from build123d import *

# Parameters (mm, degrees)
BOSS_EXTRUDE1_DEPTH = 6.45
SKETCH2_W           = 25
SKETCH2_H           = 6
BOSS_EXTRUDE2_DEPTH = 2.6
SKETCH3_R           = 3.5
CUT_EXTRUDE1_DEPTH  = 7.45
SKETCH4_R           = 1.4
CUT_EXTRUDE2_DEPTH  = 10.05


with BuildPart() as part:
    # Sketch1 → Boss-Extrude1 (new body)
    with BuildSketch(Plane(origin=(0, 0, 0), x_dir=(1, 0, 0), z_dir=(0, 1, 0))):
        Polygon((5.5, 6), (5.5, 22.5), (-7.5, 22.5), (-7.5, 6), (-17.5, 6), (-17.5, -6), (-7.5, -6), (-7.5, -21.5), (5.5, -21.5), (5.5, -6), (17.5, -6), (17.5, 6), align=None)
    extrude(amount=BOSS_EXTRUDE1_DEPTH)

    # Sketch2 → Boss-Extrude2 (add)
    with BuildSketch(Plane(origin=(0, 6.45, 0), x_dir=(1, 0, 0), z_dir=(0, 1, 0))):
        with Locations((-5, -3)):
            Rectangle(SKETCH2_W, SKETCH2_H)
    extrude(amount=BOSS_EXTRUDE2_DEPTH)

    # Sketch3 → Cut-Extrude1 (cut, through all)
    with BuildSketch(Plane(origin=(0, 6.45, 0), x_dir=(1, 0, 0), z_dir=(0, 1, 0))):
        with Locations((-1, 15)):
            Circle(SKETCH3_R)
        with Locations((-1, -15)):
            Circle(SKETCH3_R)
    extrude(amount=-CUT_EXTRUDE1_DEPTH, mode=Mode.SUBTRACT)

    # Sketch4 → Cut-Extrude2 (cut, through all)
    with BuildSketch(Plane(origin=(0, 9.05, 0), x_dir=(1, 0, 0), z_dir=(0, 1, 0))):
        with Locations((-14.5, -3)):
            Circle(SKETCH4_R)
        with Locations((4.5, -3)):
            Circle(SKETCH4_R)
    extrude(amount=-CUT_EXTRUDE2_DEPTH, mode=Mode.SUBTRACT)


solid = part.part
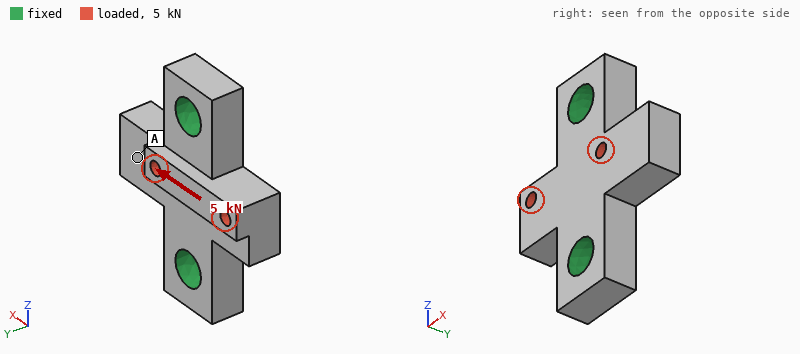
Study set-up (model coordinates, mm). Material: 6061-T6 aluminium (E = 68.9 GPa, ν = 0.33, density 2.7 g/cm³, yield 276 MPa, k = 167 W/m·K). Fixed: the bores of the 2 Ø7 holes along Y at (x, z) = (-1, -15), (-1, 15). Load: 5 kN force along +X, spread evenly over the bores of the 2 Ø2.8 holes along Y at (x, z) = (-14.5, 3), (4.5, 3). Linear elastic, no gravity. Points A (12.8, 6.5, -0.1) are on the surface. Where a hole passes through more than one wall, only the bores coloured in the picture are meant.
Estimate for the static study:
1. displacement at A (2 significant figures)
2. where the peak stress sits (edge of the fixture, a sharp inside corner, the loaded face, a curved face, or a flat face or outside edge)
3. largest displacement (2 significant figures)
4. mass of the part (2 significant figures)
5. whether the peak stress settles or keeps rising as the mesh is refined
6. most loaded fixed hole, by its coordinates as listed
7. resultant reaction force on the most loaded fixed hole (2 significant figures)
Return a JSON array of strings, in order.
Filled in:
["25 µm", "edge of the fixture", "41 µm", "14 g", "keeps rising", "(-1, 15)", "3.2 kN"]
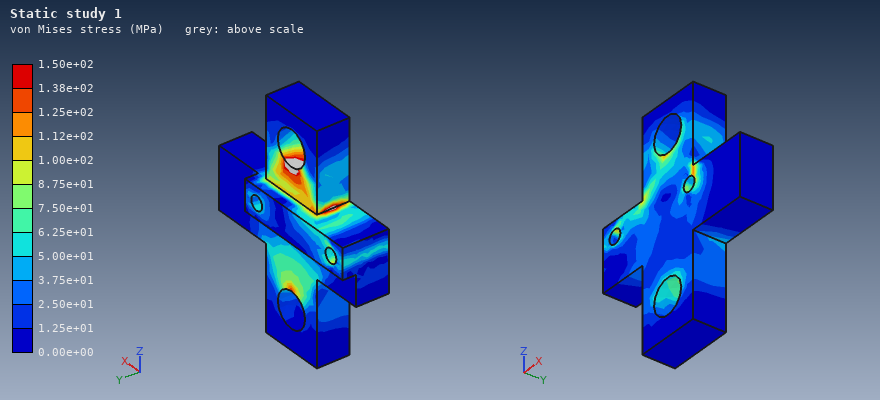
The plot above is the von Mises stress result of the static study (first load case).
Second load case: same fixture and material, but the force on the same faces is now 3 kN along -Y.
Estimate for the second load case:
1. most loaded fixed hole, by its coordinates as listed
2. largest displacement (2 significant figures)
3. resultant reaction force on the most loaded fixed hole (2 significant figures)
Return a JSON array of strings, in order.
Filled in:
["(-1, 15)", "96 µm", "2.0 kN"]
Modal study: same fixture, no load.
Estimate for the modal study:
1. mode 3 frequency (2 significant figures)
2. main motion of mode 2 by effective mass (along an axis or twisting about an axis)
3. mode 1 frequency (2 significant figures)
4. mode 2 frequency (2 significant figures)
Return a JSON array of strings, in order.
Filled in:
["29 kHz", "along Y", "12 kHz", "18 kHz"]
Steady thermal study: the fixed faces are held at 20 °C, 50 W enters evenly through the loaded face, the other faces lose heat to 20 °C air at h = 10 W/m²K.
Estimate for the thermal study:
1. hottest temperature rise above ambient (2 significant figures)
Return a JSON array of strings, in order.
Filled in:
["36 K"]
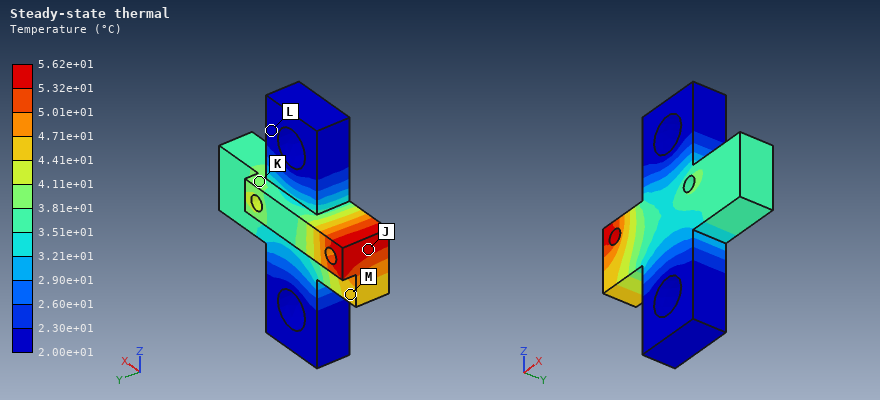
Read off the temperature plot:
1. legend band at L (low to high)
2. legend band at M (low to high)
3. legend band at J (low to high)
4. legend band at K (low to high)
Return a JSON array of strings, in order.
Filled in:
["2.00e+01 to 2.30e+01 °C", "4.41e+01 to 4.71e+01 °C", "5.32e+01 to 5.62e+01 °C", "3.81e+01 to 4.11e+01 °C"]
